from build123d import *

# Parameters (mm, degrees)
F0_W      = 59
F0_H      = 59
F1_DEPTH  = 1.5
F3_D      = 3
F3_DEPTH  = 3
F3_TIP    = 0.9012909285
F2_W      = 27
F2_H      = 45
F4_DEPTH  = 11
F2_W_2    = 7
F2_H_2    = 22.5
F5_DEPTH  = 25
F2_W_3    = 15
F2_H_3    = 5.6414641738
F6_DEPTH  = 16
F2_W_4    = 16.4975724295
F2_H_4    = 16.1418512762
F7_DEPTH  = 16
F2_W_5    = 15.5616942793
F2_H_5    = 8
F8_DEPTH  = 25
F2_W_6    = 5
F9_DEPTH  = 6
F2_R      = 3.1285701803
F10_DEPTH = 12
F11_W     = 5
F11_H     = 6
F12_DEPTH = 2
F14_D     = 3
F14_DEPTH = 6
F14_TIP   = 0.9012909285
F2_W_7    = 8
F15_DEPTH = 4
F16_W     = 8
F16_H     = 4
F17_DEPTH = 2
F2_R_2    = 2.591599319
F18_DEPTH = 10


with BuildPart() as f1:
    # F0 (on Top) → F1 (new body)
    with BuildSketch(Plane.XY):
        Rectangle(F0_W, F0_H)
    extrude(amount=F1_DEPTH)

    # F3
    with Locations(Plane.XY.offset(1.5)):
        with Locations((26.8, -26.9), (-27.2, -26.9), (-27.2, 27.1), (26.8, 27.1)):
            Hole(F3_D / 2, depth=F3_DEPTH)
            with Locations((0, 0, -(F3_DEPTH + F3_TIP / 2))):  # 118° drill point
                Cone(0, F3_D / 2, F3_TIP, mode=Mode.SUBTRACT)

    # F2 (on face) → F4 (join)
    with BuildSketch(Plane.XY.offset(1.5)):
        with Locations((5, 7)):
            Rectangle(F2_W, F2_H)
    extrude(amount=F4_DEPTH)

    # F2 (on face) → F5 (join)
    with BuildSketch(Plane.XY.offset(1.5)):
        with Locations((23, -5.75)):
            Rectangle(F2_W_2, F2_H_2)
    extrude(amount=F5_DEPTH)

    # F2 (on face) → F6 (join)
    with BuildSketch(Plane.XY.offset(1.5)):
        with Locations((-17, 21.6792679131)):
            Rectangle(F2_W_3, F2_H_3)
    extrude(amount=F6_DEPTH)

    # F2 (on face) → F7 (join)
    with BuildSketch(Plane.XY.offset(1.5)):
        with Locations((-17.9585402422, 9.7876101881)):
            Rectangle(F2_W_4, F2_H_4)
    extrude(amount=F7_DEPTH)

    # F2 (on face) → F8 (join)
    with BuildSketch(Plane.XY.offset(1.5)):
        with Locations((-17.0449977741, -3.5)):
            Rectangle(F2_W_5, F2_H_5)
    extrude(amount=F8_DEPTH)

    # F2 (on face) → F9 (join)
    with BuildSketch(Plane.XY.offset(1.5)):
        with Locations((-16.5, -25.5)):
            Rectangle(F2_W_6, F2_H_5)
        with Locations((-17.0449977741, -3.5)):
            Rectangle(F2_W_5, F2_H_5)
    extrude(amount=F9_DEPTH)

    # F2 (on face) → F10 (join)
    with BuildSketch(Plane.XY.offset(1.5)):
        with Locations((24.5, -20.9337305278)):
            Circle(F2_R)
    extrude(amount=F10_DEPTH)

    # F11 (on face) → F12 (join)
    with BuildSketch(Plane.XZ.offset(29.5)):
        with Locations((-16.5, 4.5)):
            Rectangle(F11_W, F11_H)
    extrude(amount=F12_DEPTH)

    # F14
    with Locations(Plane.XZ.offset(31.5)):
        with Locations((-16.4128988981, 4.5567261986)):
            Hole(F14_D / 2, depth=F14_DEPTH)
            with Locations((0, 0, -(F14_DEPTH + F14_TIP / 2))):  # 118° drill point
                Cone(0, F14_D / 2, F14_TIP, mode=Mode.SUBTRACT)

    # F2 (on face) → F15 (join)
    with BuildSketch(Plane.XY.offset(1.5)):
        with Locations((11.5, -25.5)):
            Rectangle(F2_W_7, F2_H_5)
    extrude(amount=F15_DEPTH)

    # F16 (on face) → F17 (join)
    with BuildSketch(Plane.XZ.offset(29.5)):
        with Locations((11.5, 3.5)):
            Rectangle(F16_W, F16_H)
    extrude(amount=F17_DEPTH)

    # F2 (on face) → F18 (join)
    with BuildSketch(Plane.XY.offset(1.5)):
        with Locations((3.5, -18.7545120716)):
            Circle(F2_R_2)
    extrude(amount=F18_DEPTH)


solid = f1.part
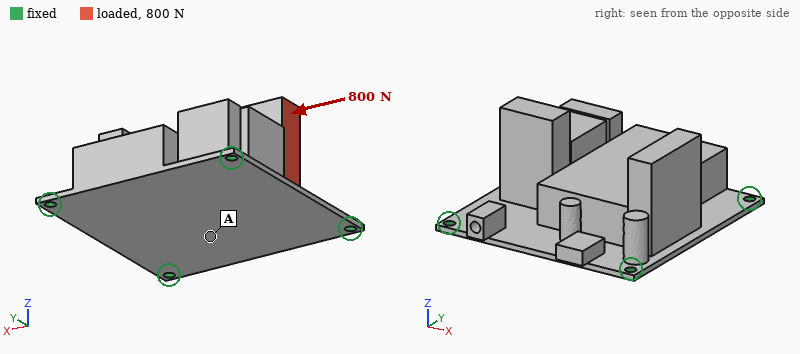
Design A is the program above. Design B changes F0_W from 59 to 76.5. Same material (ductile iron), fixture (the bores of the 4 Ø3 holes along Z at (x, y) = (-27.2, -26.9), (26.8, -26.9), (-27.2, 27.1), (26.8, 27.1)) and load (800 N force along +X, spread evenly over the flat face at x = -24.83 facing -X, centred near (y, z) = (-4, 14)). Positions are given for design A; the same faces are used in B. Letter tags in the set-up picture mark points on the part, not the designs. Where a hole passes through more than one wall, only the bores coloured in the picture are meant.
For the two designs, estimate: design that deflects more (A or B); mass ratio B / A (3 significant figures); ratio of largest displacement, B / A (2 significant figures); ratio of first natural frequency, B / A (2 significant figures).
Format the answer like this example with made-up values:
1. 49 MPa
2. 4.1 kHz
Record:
1. A
2. 1.05
3. 0.91
4. 1.0
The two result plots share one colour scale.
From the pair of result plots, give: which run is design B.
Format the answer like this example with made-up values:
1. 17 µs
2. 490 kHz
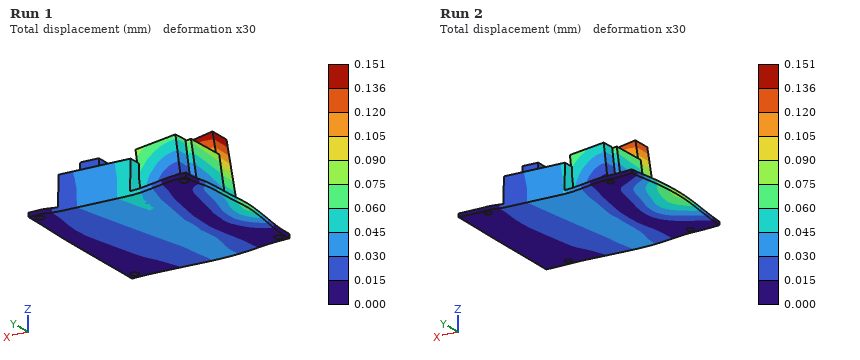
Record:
1. Run 2
